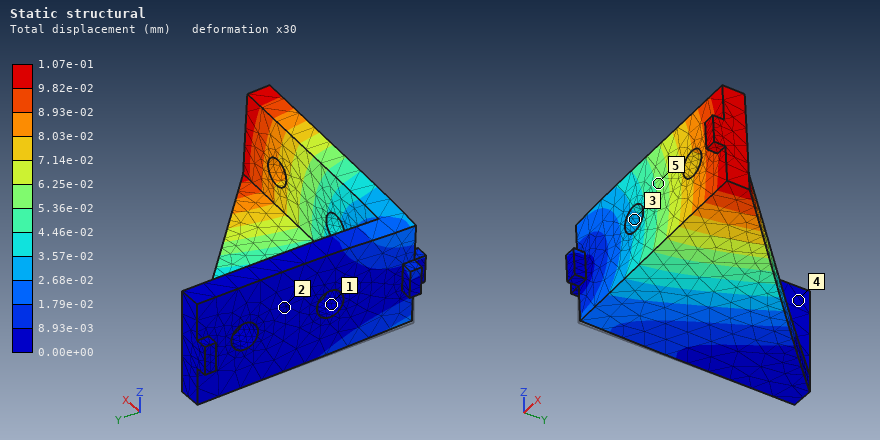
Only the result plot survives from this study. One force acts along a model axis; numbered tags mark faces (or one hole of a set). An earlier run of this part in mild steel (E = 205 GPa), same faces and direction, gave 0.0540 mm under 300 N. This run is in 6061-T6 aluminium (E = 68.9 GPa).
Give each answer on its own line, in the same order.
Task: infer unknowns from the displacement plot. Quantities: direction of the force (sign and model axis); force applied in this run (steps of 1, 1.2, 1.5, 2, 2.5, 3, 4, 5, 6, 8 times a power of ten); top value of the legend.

+Z
200 N
1.07e-01 mm
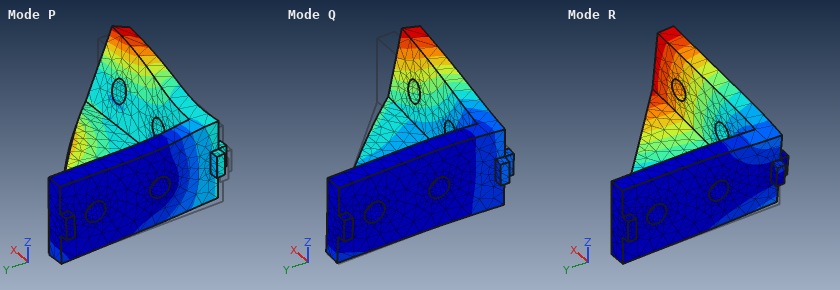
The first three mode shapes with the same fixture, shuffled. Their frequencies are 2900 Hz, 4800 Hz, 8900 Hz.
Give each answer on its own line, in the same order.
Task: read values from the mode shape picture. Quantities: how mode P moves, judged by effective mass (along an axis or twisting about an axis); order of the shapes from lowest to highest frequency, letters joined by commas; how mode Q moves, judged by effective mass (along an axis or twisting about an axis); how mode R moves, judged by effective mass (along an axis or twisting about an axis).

along X
R, Q, P
along Y
along Z
